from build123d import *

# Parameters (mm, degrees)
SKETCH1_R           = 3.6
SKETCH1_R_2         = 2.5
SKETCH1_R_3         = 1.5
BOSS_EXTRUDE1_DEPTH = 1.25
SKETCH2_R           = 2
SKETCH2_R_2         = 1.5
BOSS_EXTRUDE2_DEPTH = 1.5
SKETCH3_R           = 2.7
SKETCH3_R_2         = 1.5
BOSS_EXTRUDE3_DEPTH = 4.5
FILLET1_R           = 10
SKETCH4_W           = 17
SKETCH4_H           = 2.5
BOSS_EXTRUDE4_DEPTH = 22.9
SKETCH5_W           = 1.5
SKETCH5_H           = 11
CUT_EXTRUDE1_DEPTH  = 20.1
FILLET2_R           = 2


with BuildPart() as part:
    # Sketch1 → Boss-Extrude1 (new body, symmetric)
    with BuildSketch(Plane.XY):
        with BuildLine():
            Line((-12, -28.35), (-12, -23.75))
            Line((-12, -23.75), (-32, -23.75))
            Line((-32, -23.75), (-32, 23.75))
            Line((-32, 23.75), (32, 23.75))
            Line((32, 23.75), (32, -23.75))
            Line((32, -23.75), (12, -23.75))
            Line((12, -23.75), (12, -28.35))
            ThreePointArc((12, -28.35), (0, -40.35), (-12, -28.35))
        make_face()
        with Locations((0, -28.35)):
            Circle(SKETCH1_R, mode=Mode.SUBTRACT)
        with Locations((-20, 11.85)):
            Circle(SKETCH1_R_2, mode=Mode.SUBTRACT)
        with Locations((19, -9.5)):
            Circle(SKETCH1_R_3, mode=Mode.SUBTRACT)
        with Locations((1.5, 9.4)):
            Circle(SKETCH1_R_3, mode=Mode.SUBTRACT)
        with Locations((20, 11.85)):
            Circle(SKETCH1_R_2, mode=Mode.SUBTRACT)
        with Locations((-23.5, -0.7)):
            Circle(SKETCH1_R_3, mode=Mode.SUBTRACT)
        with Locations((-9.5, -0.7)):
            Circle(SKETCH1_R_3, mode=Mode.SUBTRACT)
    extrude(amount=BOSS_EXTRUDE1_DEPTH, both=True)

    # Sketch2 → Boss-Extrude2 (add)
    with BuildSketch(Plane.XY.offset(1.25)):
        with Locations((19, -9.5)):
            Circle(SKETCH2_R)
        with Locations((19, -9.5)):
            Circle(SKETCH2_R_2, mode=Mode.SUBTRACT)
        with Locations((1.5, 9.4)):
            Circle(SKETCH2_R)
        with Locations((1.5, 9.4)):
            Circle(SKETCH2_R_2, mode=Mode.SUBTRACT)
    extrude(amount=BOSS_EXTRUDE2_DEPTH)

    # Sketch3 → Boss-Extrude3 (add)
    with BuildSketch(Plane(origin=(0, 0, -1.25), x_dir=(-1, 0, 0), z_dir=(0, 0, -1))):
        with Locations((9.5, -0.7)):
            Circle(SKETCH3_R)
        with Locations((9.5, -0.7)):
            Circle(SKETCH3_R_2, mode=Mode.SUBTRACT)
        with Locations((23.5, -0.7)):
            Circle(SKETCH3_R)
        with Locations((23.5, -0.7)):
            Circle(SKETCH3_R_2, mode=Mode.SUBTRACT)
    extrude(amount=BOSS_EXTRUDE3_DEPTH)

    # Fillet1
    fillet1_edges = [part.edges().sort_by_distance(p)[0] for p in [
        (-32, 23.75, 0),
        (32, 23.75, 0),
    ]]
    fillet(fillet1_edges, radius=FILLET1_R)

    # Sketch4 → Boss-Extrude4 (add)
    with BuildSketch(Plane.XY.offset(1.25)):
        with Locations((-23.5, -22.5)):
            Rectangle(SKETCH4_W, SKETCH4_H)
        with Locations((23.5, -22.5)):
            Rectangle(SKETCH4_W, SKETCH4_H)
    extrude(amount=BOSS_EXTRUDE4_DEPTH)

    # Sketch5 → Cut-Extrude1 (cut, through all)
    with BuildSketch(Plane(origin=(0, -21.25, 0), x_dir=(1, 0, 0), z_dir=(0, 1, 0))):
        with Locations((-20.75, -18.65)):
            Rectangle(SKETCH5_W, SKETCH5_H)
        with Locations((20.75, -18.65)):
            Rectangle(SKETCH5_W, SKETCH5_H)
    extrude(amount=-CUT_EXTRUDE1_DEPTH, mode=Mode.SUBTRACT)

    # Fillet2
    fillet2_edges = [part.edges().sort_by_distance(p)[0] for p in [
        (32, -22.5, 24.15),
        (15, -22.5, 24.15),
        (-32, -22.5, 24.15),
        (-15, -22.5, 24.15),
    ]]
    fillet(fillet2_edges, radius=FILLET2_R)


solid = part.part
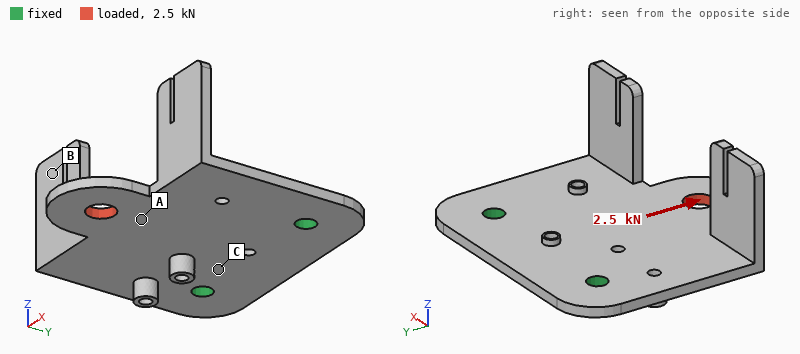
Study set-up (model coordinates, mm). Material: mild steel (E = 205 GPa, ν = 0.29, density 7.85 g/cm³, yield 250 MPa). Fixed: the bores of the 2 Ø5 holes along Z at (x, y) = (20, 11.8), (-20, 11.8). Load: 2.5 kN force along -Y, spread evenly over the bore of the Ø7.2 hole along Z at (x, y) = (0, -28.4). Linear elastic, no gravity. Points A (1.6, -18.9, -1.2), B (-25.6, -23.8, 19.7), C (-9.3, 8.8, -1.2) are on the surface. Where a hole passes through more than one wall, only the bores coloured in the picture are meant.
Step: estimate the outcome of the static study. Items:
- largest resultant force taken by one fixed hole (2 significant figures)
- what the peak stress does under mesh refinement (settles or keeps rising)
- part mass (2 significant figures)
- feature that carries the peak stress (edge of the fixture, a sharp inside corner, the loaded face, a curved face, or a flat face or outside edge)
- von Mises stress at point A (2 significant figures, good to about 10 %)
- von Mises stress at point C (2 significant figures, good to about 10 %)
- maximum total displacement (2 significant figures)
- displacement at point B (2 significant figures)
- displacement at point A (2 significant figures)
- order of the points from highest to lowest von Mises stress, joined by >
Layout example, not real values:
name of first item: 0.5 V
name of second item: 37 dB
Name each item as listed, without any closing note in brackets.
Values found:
largest resultant force taken by one fixed hole: 1.3 kN
what the peak stress does under mesh refinement: keeps rising
part mass: 79 g
feature that carries the peak stress: a sharp inside corner
von Mises stress at point A: 37 MPa
von Mises stress at point C: 17 MPa
maximum total displacement: 8.8 µm
displacement at point B: 2.3 µm
displacement at point A: 5.3 µm
order of the points from highest to lowest von Mises stress, joined by >: A > C > B
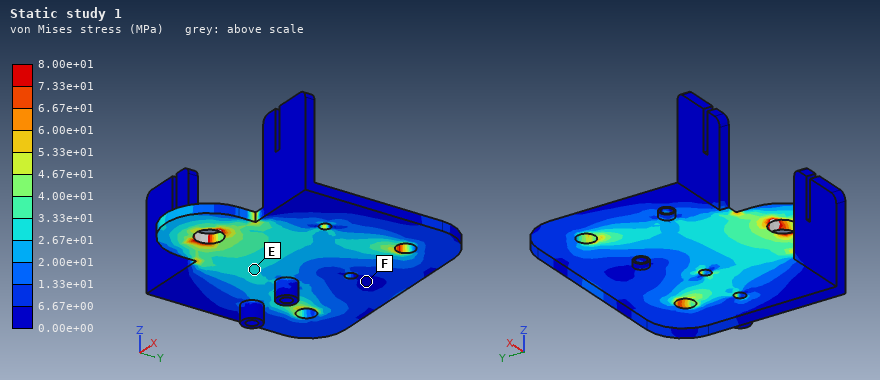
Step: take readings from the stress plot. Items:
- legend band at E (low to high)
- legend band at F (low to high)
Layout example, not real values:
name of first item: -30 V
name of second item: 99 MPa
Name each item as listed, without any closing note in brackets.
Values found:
legend band at E: 2.67e+01 to 3.33e+01 MPa
legend band at F: 0.00e+00 to 6.67e+00 MPa
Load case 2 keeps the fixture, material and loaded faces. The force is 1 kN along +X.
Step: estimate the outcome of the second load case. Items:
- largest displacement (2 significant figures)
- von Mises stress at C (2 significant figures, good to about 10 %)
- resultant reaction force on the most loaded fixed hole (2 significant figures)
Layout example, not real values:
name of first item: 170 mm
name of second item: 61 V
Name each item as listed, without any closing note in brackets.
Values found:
largest displacement: 11 µm
von Mises stress at C: 13 MPa
resultant reaction force on the most loaded fixed hole: 1.1 kN
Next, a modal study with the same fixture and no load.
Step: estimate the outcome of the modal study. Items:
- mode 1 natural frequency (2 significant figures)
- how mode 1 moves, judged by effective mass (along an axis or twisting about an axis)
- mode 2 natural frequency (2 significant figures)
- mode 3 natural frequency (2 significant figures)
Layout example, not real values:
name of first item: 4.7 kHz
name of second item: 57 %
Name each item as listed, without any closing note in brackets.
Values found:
mode 1 natural frequency: 850 Hz
how mode 1 moves, judged by effective mass: along Z
mode 2 natural frequency: 1400 Hz
mode 3 natural frequency: 2200 Hz
